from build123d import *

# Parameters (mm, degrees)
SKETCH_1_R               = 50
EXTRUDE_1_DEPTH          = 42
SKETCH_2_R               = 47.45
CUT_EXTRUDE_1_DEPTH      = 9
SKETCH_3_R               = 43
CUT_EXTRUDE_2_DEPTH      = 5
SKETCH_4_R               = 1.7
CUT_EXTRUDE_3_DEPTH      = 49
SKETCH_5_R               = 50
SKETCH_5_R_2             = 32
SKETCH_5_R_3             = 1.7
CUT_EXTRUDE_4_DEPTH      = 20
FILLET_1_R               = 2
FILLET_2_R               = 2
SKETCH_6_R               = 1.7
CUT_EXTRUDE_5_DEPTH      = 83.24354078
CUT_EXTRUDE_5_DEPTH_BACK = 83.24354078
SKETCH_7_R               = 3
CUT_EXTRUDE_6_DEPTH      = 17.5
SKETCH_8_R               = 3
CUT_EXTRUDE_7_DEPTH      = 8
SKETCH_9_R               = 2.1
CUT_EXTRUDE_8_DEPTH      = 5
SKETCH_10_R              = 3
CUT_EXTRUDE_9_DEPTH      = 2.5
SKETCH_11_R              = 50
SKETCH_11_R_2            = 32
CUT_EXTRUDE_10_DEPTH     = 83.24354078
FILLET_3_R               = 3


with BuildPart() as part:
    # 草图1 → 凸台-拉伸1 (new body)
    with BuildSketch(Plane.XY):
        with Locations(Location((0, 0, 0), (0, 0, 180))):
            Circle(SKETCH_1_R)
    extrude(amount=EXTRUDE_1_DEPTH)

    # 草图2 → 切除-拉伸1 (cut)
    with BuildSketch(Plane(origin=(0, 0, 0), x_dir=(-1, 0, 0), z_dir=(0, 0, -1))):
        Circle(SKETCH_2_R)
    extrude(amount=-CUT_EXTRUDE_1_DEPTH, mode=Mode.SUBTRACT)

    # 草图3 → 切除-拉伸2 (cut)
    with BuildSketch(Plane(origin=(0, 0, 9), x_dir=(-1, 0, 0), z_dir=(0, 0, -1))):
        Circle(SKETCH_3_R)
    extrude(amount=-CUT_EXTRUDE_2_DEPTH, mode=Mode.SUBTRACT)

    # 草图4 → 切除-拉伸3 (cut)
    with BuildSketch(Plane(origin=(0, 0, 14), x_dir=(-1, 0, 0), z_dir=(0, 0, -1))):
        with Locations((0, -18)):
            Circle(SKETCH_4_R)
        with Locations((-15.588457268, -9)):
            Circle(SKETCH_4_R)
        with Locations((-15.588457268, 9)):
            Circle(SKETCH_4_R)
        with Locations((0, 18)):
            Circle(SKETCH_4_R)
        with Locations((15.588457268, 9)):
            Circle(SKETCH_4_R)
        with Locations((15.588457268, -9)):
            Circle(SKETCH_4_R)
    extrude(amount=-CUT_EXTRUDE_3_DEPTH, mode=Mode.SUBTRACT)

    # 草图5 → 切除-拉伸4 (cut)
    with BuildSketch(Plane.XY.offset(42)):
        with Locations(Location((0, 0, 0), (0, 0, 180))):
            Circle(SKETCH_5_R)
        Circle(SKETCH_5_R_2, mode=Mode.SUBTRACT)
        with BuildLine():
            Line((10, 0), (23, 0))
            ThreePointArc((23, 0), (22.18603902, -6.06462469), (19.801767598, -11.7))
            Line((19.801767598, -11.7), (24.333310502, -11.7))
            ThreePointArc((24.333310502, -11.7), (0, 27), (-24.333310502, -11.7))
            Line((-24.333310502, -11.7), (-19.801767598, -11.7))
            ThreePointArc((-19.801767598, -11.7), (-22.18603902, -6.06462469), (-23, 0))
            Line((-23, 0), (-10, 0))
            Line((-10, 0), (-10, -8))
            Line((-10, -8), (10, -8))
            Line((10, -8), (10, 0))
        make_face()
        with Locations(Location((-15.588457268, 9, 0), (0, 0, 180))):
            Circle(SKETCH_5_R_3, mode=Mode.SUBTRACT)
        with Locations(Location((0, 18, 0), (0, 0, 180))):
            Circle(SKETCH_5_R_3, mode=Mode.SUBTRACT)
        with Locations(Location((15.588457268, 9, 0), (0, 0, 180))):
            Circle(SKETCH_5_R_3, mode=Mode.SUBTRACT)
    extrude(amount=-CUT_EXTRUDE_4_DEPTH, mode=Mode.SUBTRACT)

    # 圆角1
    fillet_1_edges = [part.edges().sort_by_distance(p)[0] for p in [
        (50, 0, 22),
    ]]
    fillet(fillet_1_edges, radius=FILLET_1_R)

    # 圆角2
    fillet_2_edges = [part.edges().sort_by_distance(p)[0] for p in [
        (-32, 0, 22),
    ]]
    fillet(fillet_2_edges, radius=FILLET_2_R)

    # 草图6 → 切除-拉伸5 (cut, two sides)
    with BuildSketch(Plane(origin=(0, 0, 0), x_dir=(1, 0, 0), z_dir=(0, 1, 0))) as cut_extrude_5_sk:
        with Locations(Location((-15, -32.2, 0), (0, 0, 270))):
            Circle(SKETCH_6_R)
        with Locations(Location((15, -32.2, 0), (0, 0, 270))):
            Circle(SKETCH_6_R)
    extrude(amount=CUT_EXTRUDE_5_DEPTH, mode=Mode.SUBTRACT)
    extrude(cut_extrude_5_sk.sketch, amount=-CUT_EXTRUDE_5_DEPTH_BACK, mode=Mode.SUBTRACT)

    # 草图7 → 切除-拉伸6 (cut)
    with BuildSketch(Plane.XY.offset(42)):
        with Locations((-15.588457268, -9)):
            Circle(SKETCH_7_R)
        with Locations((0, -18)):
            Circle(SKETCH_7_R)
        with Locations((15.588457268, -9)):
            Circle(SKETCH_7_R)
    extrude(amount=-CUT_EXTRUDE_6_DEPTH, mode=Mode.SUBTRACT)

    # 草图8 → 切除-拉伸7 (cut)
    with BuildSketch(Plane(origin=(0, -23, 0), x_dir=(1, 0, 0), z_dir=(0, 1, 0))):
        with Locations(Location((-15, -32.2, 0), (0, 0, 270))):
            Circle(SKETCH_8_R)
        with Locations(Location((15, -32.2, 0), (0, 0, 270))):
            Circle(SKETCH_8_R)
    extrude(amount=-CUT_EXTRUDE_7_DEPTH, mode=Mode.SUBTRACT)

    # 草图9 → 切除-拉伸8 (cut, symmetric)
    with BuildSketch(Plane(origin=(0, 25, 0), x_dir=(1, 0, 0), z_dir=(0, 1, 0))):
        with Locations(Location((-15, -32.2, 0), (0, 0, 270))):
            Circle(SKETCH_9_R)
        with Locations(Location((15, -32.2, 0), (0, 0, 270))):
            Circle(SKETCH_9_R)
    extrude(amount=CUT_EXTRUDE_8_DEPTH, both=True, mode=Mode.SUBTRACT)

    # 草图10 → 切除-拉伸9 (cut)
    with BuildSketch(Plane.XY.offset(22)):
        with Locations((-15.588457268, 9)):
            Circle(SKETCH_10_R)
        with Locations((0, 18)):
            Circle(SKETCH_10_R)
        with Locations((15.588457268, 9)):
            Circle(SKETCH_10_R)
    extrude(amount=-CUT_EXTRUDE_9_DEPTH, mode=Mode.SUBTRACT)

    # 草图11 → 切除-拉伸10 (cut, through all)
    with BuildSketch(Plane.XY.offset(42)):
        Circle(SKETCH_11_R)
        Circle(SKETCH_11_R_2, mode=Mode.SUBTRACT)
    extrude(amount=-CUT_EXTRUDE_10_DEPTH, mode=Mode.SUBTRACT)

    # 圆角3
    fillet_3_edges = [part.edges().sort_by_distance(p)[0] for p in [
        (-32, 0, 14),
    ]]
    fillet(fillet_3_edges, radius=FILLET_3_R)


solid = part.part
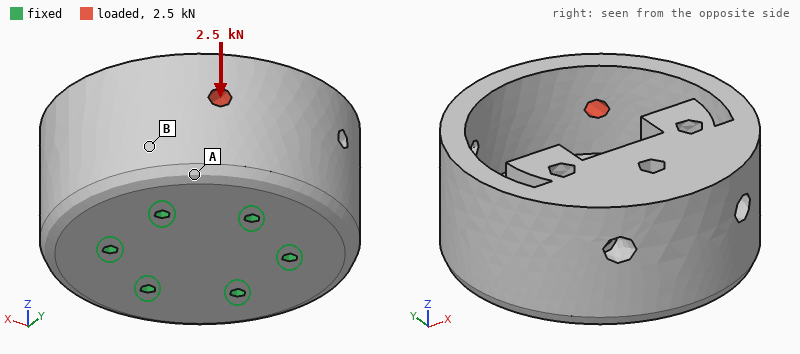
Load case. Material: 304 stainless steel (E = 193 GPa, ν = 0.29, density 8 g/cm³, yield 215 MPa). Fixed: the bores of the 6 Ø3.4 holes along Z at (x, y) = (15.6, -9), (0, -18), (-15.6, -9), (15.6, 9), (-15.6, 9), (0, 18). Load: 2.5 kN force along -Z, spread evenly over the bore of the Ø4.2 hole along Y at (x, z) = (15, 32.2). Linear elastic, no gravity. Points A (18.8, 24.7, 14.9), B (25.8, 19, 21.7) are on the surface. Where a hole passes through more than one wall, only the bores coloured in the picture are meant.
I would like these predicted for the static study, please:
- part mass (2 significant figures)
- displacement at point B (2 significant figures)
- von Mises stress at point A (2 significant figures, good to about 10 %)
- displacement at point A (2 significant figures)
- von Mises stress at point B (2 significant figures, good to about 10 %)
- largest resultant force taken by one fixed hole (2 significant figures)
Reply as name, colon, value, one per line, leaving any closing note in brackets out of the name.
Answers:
part mass: 470 g
displacement at point B: 7.0 µm
von Mises stress at point A: 8.8 MPa
displacement at point A: 8.4 µm
von Mises stress at point B: 23 MPa
largest resultant force taken by one fixed hole: 1.6 kN
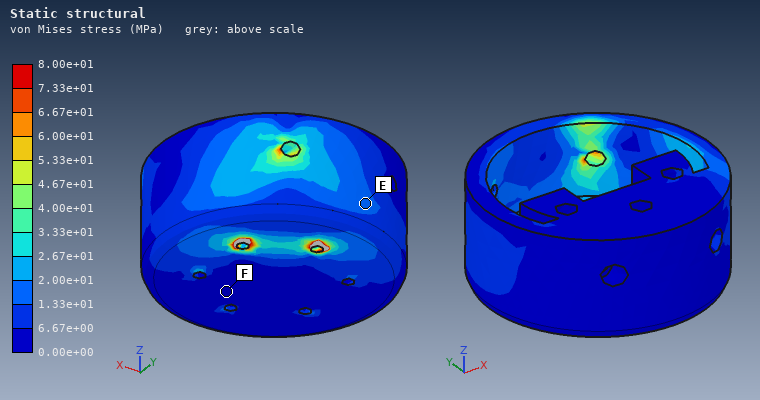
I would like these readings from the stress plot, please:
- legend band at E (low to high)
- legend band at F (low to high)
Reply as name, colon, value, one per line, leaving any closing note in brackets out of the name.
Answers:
legend band at E: 1.33e+01 to 2.00e+01 MPa
legend band at F: 0.00e+00 to 6.67e+00 MPa
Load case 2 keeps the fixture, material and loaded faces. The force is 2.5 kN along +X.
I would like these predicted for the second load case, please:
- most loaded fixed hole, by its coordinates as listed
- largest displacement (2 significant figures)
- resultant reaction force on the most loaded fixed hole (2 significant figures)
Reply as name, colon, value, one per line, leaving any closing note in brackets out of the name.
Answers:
most loaded fixed hole, by its coordinates as listed: (0, 18)
largest displacement: 16 µm
resultant reaction force on the most loaded fixed hole: 1.5 kN
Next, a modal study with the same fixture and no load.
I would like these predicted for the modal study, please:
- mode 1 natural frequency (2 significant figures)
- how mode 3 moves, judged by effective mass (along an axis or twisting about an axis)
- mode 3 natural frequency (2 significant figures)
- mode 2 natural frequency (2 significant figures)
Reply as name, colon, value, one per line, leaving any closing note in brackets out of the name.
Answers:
mode 1 natural frequency: 9700 Hz
how mode 3 moves, judged by effective mass: along Y
mode 3 natural frequency: 12 kHz
mode 2 natural frequency: 9800 Hz
